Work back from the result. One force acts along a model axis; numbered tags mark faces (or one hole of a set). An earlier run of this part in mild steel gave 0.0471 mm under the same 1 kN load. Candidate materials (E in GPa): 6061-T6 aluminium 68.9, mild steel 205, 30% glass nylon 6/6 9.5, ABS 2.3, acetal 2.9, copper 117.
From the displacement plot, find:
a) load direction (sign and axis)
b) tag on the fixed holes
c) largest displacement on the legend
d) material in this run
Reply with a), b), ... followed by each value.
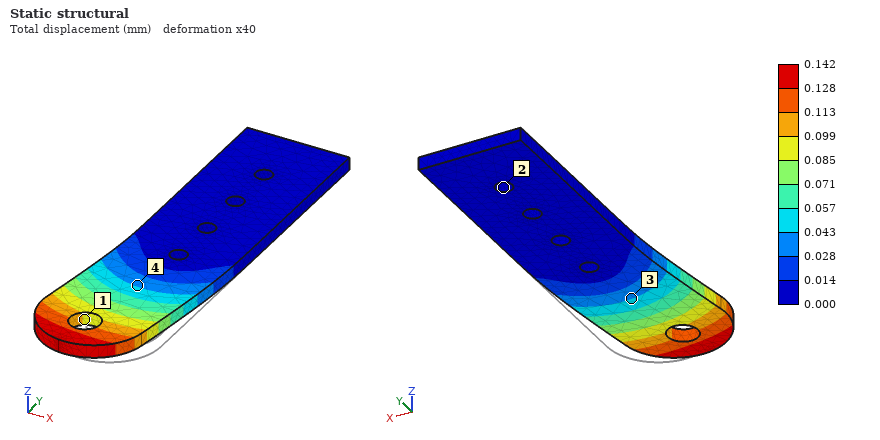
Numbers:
a) -X
b) 2
c) 0.142 mm
d) 6061-T6 aluminium
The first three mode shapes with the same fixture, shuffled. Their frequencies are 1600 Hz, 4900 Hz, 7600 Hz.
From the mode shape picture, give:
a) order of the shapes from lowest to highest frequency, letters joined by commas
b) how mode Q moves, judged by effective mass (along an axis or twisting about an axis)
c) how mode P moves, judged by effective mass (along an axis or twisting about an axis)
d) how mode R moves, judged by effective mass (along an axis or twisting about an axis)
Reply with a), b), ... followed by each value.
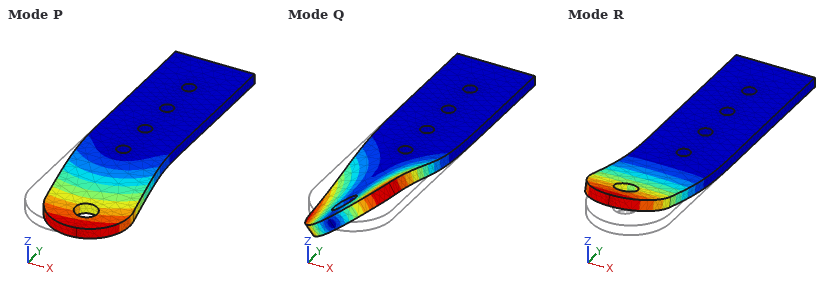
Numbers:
a) R, Q, P
b) twisting about Y
c) along X
d) along Z
